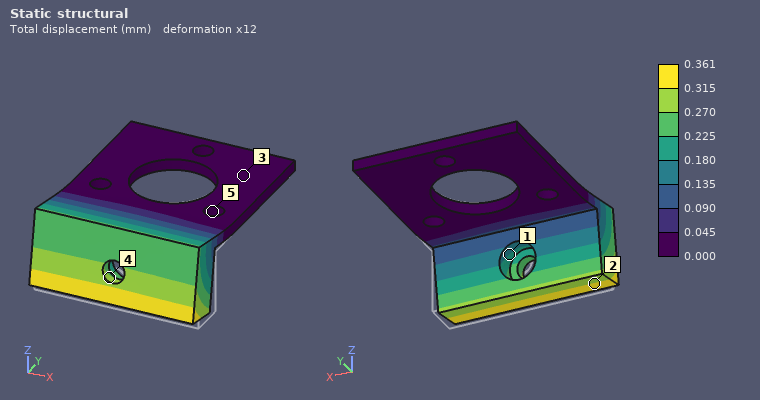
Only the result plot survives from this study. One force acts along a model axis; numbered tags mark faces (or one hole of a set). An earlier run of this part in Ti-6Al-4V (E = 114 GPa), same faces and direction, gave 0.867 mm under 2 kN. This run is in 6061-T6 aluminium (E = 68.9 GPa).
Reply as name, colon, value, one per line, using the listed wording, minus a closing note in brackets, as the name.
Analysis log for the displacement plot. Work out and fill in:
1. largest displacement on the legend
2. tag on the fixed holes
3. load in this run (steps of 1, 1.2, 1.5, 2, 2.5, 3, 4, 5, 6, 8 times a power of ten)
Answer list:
largest displacement on the legend: 0.361 mm
tag on the fixed holes: 5
load in this run: 500 N
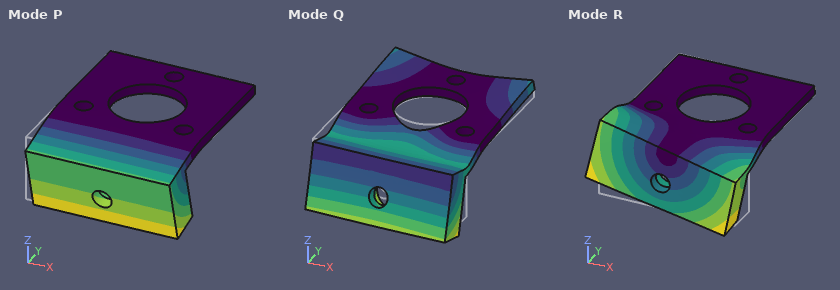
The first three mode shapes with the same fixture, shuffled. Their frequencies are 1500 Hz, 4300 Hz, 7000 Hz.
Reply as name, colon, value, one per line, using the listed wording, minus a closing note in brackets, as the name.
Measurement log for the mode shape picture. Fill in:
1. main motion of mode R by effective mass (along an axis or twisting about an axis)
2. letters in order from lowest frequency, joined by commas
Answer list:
main motion of mode R by effective mass: along X
letters in order from lowest frequency, joined by commas: P, R, Q
